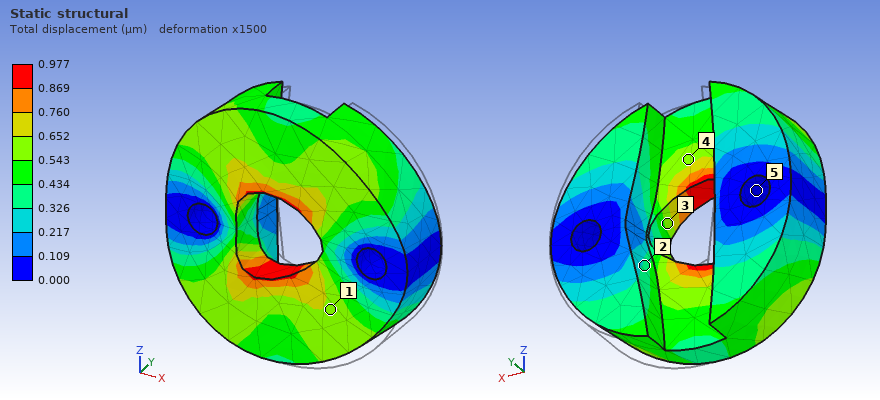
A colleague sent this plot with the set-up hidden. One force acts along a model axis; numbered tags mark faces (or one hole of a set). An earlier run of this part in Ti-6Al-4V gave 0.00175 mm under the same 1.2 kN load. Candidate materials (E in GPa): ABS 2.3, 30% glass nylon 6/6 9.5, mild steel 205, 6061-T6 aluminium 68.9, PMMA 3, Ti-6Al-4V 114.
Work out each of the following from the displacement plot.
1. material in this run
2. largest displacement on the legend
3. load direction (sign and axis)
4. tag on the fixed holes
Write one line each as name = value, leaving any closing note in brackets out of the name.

material in this run = mild steel
largest displacement on the legend = 0.977 µm
load direction = -X
tag on the fixed holes = 5
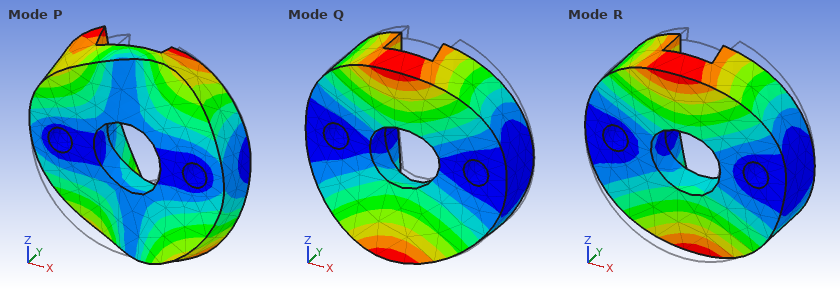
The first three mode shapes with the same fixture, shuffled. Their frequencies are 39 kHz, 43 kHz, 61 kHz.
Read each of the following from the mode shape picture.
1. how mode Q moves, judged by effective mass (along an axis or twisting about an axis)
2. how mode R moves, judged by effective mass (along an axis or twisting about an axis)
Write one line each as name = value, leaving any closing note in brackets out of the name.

how mode Q moves, judged by effective mass = along Y
how mode R moves, judged by effective mass = twisting about X
